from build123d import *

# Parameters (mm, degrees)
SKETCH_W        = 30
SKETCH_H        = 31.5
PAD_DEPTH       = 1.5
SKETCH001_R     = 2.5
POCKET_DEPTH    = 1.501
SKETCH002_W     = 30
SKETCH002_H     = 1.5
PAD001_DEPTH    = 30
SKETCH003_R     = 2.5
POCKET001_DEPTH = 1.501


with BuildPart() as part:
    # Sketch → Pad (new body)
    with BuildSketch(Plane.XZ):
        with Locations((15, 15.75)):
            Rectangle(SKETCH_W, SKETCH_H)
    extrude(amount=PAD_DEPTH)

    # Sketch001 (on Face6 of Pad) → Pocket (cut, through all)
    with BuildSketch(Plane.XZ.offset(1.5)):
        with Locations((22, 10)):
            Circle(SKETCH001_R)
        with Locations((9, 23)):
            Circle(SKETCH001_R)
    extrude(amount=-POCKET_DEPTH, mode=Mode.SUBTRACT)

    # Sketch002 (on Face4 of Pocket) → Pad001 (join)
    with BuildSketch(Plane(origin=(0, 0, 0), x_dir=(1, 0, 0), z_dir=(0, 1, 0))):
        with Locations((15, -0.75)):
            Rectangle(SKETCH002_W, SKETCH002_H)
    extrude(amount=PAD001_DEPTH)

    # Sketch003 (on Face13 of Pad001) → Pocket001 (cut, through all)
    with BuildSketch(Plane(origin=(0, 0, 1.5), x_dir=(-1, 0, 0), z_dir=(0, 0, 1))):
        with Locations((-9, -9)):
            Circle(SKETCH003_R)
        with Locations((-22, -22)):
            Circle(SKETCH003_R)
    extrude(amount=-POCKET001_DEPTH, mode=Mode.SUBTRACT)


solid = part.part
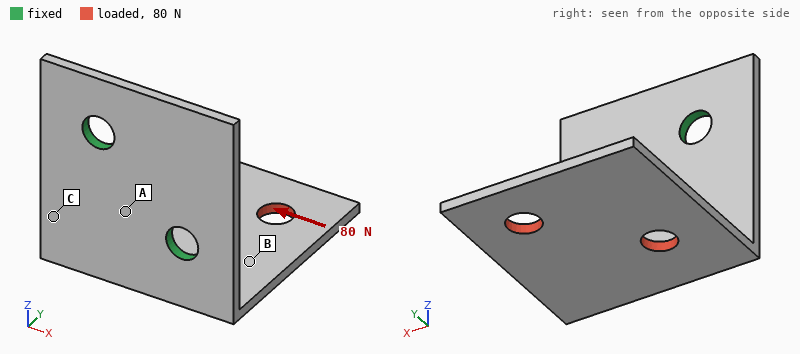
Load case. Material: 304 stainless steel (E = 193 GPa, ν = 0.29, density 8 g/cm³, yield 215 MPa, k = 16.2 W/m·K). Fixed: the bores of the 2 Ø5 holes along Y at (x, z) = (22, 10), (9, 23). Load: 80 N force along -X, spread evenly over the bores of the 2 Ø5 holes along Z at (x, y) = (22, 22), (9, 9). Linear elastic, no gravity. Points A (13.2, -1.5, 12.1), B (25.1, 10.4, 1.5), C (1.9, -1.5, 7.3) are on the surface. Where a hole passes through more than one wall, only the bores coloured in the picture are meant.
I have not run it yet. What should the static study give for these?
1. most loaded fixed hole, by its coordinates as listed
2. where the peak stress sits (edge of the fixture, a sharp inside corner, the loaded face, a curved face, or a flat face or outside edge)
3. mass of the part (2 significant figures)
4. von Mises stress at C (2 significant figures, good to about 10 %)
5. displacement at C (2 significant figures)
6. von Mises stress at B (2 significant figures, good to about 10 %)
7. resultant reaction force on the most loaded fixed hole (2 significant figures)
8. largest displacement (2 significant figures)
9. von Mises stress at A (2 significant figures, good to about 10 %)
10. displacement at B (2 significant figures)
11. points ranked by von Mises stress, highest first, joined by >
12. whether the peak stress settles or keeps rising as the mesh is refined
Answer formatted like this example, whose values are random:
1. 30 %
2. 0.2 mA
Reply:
1. (22, 10)
2. edge of the fixture
3. 21 g
4. 29 MPa
5. 0.038 mm
6. 14 MPa
7. 92 N
8. 0.13 mm
9. 48 MPa
10. 0.038 mm
11. A > C > B
12. keeps rising
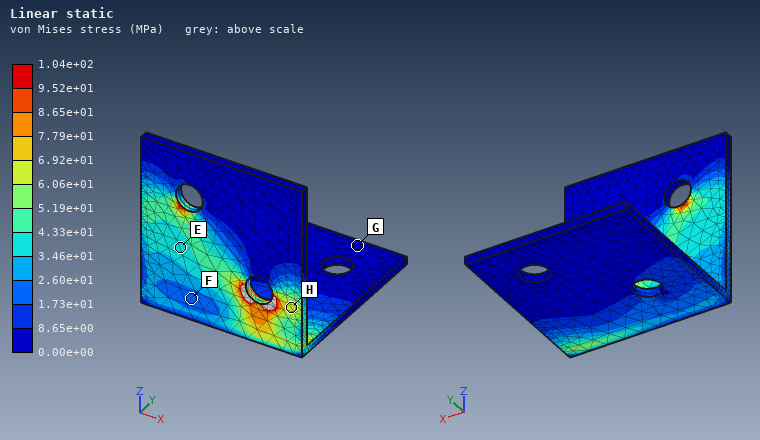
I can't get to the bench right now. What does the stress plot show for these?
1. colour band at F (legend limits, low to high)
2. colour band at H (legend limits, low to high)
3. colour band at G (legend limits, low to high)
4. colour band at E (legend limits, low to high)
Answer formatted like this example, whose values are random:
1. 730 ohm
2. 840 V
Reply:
1. 1.73e+01 to 2.60e+01 MPa
2. 6.06e+01 to 6.92e+01 MPa
3. 0.00e+00 to 8.65e+00 MPa
4. 3.46e+01 to 4.33e+01 MPa
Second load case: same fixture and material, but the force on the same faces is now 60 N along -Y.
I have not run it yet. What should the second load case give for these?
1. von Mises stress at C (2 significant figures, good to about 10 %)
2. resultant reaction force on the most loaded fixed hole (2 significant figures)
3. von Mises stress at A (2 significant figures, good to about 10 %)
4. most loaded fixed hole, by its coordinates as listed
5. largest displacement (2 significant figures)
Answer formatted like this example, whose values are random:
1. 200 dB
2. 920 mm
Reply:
1. 13 MPa
2. 59 N
3. 23 MPa
4. (22, 10)
5. 68 µm
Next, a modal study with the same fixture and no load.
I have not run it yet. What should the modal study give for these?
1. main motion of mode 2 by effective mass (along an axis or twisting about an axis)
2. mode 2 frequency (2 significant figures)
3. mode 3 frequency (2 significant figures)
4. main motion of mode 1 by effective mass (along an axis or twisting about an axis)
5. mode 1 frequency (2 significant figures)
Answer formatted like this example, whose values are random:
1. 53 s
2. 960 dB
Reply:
1. along X
2. 1500 Hz
3. 2900 Hz
4. along Z
5. 860 Hz
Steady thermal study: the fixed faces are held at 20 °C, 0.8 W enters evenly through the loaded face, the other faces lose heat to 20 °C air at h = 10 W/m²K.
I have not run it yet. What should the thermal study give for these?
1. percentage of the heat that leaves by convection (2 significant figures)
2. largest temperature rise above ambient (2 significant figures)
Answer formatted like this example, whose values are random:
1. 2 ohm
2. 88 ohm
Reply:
1. 42 %
2. 23 K
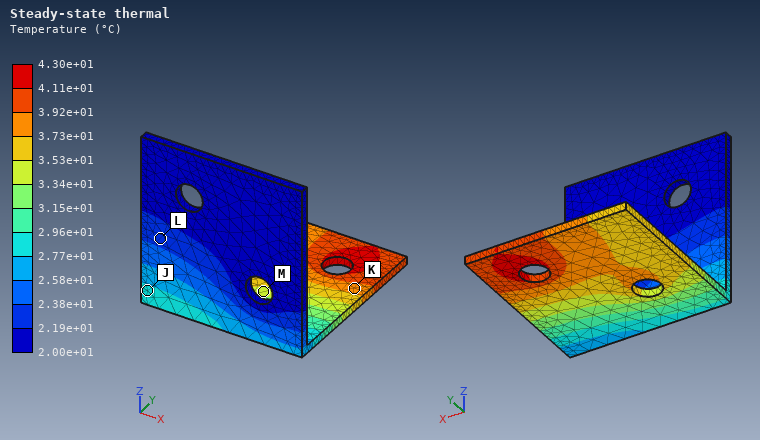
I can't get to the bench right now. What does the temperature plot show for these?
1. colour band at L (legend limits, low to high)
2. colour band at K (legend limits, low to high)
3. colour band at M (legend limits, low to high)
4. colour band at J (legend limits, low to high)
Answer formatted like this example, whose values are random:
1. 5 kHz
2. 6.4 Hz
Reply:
1. 2.19e+01 to 2.38e+01 °C
2. 3.73e+01 to 3.92e+01 °C
3. 3.34e+01 to 3.53e+01 °C
4. 2.77e+01 to 2.96e+01 °C
